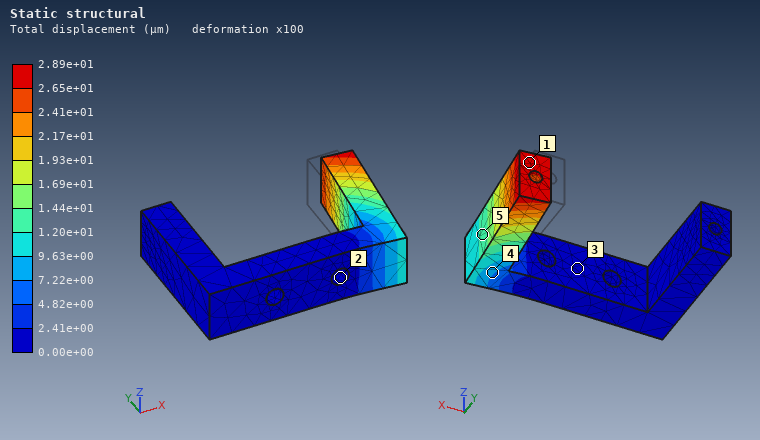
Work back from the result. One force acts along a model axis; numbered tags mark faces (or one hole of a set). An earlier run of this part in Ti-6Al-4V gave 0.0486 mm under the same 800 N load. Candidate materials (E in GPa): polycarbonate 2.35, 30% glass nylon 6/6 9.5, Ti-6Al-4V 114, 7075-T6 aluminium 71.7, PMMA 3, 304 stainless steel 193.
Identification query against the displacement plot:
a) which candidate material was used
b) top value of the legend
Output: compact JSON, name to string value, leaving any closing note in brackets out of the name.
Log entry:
{"which candidate material was used": "304 stainless steel", "top value of the legend": "2.89e+01 µm"}
